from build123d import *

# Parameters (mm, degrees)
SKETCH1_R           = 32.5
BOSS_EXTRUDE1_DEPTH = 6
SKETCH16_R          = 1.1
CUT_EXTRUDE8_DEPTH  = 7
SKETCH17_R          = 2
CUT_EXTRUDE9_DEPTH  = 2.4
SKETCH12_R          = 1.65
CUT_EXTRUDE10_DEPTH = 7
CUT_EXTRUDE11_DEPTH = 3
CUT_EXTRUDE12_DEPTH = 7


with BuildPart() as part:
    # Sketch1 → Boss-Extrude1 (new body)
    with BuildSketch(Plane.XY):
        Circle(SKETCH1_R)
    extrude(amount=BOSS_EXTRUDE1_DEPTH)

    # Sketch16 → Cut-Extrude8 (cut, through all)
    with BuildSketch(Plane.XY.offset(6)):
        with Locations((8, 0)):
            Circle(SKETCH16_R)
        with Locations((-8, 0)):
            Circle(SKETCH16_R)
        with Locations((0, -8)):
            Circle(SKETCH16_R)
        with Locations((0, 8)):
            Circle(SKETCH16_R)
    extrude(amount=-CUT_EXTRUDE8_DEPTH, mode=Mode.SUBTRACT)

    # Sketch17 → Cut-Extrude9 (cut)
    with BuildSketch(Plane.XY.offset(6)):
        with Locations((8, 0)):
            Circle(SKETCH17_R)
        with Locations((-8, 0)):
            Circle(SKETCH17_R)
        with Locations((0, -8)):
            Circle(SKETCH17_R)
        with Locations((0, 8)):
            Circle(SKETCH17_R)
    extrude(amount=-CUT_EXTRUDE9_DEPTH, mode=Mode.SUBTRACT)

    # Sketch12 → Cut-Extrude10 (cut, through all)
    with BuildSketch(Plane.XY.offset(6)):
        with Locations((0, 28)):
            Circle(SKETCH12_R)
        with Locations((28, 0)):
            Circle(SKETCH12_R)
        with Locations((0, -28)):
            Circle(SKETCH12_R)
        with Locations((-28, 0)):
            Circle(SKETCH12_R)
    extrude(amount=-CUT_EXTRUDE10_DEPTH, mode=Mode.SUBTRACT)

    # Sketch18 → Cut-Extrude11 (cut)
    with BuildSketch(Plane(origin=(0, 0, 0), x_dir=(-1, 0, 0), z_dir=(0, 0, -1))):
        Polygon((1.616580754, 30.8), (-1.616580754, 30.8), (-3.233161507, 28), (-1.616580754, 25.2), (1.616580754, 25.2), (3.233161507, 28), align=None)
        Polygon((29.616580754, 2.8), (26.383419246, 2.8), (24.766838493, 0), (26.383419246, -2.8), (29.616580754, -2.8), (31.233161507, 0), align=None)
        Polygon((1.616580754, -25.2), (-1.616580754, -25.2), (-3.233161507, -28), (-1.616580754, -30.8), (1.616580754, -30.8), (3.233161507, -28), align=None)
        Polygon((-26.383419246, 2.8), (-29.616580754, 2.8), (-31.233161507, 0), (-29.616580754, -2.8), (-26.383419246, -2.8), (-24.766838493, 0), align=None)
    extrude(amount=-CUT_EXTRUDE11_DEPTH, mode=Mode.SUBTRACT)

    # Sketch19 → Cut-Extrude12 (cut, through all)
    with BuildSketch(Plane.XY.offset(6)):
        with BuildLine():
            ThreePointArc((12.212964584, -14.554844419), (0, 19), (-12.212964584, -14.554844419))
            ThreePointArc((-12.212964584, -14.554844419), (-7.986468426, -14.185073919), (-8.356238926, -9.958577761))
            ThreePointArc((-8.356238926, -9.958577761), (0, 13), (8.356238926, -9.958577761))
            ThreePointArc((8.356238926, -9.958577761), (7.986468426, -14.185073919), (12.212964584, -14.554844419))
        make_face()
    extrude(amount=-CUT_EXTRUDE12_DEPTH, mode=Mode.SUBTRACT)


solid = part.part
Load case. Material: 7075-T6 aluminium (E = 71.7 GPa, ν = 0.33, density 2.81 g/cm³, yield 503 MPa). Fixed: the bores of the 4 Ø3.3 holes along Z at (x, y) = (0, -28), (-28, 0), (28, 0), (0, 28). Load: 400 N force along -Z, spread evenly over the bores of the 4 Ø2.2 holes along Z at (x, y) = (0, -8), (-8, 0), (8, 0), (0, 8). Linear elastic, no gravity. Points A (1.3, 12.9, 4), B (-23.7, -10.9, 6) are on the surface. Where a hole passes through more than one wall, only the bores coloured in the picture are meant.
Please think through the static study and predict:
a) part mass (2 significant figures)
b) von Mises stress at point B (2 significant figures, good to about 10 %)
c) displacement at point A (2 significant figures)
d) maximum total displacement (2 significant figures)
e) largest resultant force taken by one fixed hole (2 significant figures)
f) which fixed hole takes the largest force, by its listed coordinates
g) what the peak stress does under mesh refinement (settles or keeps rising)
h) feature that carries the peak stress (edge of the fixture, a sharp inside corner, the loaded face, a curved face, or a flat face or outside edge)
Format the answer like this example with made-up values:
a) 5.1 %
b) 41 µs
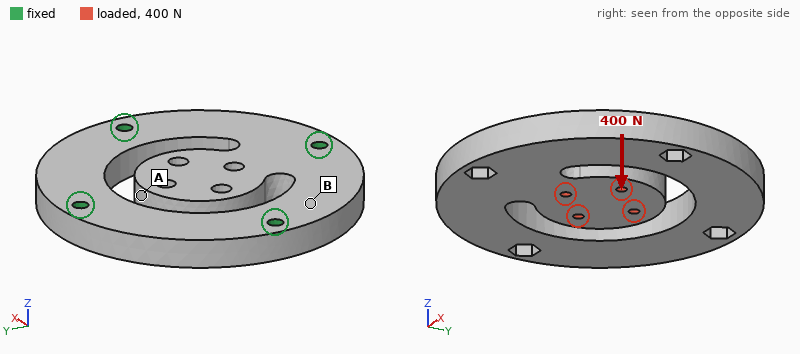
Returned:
a) 46 g
b) 20 MPa
c) 0.22 mm
d) 0.22 mm
e) 370 N
f) (0, -28)
g) keeps rising
h) edge of the fixture
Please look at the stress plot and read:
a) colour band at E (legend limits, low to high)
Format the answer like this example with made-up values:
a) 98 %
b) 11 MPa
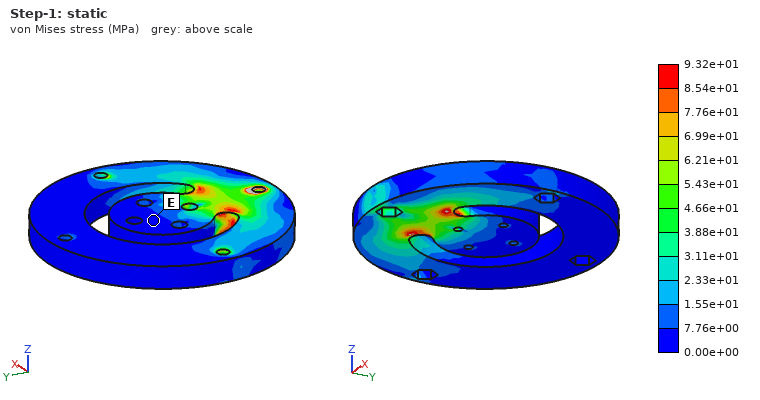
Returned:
a) 0.00e+00 to 7.76e+00 MPa
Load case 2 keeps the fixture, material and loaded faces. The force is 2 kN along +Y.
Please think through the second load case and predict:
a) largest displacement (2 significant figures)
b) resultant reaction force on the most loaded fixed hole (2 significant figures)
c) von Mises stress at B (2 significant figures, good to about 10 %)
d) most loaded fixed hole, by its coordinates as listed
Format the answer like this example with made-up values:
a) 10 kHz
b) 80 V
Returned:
a) 95 µm
b) 1.4 kN
c) 7.9 MPa
d) (0, -28)
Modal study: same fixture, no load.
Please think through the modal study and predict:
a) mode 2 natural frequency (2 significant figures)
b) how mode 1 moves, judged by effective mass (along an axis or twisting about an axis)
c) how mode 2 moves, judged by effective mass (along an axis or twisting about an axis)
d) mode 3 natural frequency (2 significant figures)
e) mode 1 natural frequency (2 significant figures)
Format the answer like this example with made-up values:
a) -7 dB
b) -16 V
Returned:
a) 7100 Hz
b) along Z
c) along X
d) 8500 Hz
e) 2800 Hz
